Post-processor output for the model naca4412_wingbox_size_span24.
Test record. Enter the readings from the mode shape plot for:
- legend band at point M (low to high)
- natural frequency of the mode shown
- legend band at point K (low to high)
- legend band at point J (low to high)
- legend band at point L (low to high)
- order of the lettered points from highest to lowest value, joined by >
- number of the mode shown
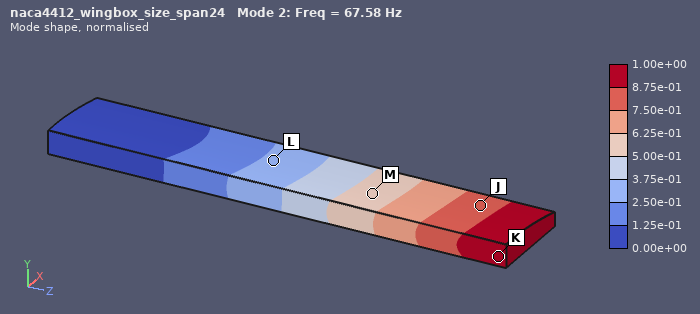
5.00e-01 to 6.25e-01
67.58 Hz
8.75e-01 to 1.00e+00
7.50e-01 to 8.75e-01
2.50e-01 to 3.75e-01
K > J > M > L
2
